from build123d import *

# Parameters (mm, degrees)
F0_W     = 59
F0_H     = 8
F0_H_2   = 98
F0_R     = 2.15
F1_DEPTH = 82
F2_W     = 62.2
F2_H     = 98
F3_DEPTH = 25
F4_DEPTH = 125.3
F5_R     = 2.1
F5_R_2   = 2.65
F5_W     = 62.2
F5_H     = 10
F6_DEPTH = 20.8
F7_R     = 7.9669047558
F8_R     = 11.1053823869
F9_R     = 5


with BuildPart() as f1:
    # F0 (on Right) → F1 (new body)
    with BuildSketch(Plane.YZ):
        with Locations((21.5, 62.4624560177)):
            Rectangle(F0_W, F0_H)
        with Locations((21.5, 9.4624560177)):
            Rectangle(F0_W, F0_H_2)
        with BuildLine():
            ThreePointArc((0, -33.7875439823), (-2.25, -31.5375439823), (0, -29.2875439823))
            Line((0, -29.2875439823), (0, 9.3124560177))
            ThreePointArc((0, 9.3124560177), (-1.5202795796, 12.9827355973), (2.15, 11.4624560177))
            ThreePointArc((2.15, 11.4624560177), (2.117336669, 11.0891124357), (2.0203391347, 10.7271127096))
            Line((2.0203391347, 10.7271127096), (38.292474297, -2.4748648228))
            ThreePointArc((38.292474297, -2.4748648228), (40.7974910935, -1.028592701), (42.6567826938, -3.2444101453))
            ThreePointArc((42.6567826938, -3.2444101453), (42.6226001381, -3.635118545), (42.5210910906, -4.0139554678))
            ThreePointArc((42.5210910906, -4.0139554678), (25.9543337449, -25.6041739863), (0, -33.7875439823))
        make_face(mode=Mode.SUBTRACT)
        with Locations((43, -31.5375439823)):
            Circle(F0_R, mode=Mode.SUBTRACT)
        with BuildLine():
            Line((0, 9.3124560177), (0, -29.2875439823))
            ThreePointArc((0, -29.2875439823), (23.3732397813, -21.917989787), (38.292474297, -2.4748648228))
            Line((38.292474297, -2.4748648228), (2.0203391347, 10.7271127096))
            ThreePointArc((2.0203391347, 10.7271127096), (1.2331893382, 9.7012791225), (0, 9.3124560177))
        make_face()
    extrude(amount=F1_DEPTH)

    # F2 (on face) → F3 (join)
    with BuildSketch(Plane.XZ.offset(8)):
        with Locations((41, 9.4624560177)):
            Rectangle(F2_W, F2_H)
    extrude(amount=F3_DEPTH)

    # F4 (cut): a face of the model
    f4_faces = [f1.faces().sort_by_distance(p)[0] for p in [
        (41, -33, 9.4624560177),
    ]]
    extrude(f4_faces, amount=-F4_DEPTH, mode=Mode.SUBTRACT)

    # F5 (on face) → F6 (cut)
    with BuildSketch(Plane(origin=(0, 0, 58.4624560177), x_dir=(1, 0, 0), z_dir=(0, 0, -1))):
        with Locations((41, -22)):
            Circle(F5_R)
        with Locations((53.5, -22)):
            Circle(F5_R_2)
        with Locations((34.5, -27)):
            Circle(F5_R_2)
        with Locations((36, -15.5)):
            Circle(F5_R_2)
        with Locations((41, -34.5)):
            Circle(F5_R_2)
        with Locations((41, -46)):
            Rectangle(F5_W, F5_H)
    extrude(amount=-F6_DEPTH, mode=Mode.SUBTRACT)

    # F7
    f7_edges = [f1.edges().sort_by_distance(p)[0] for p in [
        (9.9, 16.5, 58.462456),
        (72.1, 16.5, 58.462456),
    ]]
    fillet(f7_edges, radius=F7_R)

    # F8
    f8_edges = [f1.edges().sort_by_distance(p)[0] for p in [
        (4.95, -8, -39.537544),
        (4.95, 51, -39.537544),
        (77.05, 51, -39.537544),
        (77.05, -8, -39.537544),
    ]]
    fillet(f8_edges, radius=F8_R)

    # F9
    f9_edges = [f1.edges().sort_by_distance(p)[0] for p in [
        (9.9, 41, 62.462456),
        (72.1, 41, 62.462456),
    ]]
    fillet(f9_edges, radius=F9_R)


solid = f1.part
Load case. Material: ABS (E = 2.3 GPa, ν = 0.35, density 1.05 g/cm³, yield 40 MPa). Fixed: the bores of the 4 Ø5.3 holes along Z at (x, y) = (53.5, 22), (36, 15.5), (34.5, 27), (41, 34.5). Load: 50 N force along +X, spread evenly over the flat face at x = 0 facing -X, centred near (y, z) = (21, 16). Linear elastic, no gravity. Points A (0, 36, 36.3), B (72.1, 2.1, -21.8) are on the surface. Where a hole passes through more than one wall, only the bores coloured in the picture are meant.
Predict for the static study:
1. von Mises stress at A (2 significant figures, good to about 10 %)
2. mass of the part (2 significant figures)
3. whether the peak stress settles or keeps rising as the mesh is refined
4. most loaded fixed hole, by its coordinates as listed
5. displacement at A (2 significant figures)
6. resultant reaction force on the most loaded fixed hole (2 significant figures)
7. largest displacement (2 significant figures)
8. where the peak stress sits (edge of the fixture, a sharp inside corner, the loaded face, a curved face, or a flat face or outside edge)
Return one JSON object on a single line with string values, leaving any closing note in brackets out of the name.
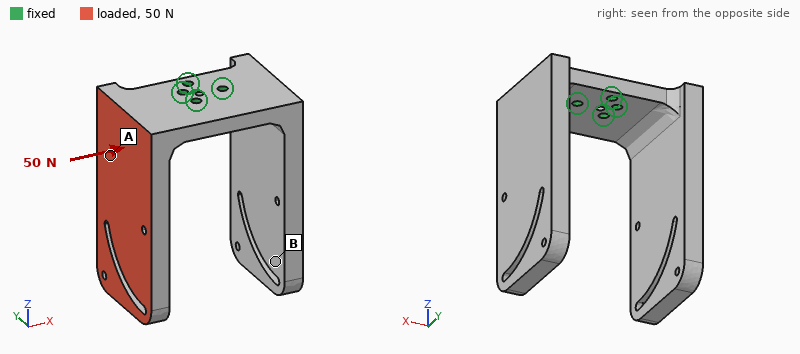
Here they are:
{"von Mises stress at A": "1.2 MPa", "mass of the part": "150 g", "whether the peak stress settles or keeps rising as the mesh is refined": "keeps rising", "most loaded fixed hole, by its coordinates as listed": "(34.5, 27)", "displacement at A": "0.44 mm", "resultant reaction force on the most loaded fixed hole": "47 N", "largest displacement": "1.6 mm", "where the peak stress sits": "edge of the fixture"}
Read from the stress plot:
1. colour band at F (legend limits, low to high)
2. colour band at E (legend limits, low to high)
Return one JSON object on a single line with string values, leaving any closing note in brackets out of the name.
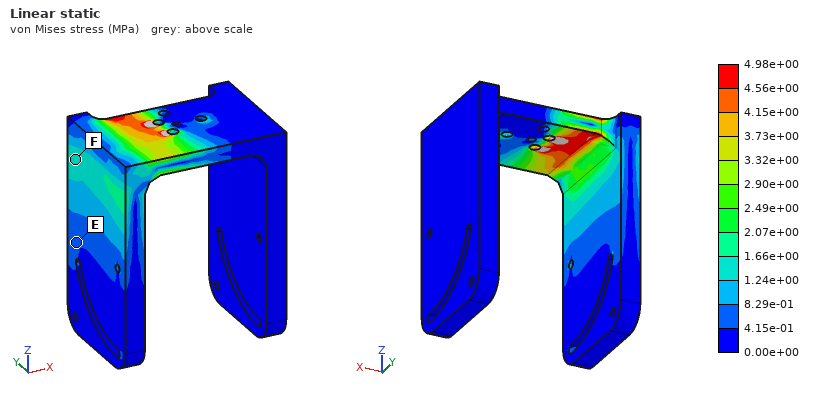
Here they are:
{"colour band at F": "1.24e+00 to 1.66e+00 MPa", "colour band at E": "4.15e-01 to 8.29e-01 MPa"}
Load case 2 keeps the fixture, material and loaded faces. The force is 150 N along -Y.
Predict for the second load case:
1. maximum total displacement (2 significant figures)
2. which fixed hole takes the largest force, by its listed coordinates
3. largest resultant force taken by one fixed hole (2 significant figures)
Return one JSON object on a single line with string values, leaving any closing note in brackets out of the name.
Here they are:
{"maximum total displacement": "1.7 mm", "which fixed hole takes the largest force, by its listed coordinates": "(36, 15.5)", "largest resultant force taken by one fixed hole": "350 N"}
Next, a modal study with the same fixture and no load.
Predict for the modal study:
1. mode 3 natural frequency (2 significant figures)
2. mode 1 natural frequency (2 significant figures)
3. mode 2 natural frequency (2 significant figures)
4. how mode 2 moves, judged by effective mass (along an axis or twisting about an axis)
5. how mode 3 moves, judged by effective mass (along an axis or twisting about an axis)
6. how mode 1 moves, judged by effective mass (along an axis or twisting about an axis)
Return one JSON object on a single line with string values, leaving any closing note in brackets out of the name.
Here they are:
{"mode 3 natural frequency": "220 Hz", "mode 1 natural frequency": "140 Hz", "mode 2 natural frequency": "150 Hz", "how mode 2 moves, judged by effective mass": "along X", "how mode 3 moves, judged by effective mass": "along Y", "how mode 1 moves, judged by effective mass": "along X"}
